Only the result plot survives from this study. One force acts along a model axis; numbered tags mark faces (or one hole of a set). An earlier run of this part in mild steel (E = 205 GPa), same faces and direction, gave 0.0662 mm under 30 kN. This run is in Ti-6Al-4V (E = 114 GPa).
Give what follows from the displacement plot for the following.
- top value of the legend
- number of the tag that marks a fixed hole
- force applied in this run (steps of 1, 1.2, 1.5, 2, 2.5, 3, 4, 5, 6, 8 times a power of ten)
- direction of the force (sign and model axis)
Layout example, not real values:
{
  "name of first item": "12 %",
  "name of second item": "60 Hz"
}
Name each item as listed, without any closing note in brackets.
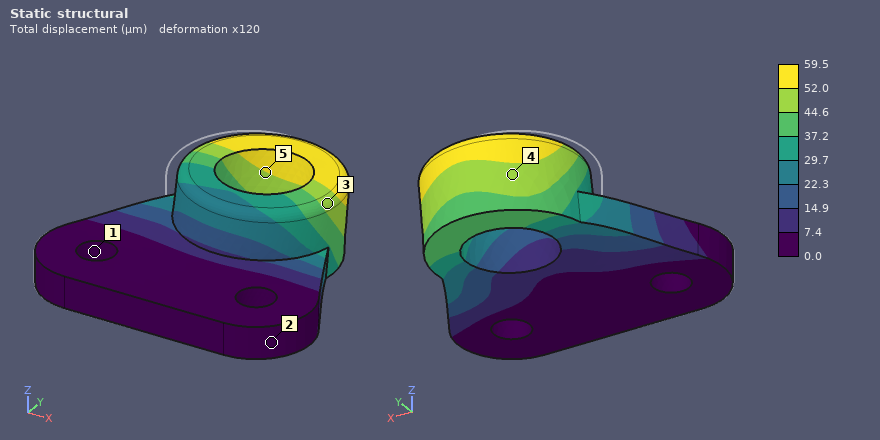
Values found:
{
  "top value of the legend": "59.5 µm",
  "number of the tag that marks a fixed hole": "1",
  "force applied in this run": "15 kN",
  "direction of the force": "+X"
}
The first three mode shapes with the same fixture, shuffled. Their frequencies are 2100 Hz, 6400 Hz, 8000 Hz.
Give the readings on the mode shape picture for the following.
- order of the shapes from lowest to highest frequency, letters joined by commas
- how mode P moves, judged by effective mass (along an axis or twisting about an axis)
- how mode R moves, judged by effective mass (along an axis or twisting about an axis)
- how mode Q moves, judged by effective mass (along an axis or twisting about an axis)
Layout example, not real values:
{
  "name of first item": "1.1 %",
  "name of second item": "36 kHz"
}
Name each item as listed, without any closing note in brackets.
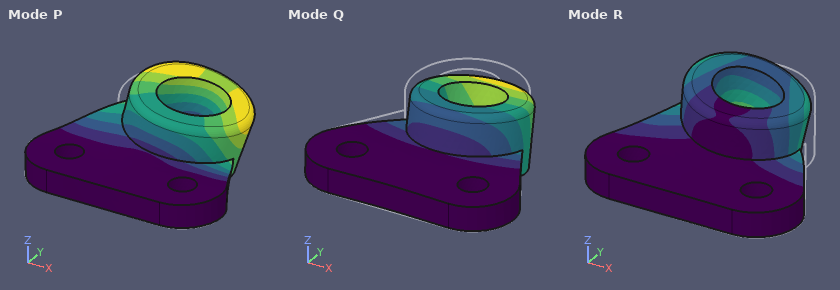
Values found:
{
  "order of the shapes from lowest to highest frequency, letters joined by commas": "Q, P, R",
  "how mode P moves, judged by effective mass": "along X",
  "how mode R moves, judged by effective mass": "along X",
  "how mode Q moves, judged by effective mass": "along Z"
}
